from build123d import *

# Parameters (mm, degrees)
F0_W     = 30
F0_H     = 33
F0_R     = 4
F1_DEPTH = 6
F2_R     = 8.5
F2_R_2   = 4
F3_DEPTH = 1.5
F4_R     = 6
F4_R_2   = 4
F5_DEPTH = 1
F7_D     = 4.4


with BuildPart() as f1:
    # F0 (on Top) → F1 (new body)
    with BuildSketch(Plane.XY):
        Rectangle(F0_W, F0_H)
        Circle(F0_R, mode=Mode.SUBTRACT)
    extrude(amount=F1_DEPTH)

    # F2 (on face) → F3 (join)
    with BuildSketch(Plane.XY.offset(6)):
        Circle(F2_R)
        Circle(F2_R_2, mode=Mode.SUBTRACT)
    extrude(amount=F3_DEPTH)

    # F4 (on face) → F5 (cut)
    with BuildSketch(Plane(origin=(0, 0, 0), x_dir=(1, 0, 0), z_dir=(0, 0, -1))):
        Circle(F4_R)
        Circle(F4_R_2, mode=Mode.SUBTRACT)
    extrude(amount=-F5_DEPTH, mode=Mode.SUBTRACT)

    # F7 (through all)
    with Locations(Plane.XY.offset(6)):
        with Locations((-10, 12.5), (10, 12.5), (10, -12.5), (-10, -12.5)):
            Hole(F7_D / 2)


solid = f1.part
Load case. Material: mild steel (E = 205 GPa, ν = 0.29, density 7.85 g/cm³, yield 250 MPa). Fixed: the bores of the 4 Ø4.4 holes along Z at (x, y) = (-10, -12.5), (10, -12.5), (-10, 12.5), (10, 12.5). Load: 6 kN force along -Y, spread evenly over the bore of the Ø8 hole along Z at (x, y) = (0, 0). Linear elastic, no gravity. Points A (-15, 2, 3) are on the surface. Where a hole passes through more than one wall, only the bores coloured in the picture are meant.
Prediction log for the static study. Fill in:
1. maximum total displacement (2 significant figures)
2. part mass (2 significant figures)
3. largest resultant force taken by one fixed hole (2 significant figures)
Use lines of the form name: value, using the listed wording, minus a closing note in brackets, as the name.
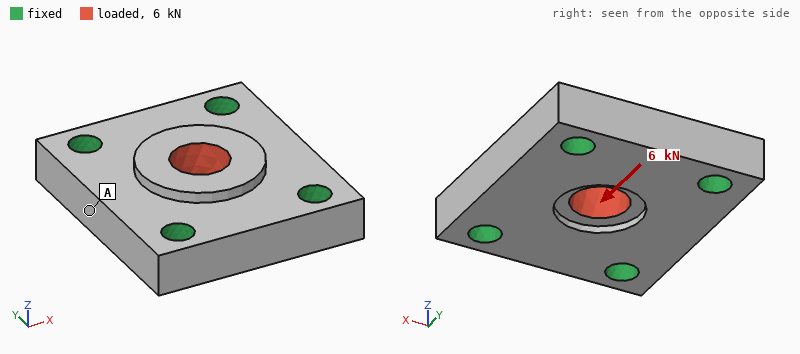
maximum total displacement: 2.7 µm
part mass: 43 g
largest resultant force taken by one fixed hole: 1.6 kN
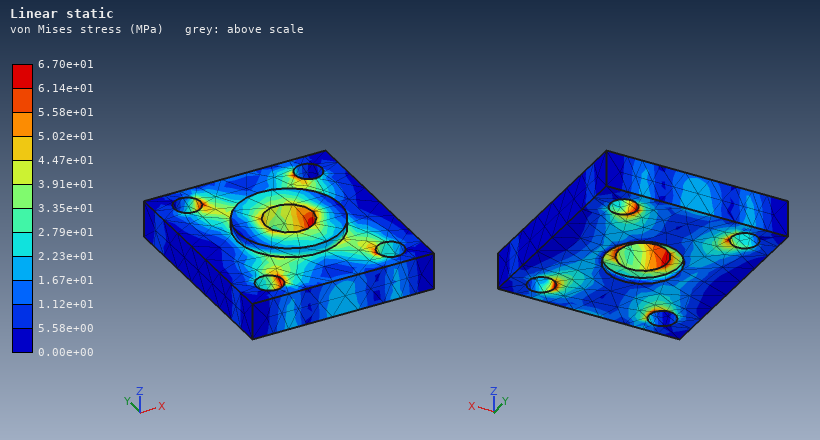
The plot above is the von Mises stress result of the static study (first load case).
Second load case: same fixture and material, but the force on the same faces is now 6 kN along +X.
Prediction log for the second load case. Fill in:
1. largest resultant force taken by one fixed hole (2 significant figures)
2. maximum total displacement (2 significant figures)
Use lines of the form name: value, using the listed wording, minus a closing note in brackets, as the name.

largest resultant force taken by one fixed hole: 1.7 kN
maximum total displacement: 3.4 µm
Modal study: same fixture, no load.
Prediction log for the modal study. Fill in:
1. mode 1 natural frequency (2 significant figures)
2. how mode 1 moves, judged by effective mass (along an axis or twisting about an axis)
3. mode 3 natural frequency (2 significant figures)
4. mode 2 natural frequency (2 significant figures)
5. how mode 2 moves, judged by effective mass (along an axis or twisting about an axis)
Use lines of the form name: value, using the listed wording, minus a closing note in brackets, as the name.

mode 1 natural frequency: 39 kHz
how mode 1 moves, judged by effective mass: along Z
mode 3 natural frequency: 56 kHz
mode 2 natural frequency: 47 kHz
how mode 2 moves, judged by effective mass: twisting about Y
